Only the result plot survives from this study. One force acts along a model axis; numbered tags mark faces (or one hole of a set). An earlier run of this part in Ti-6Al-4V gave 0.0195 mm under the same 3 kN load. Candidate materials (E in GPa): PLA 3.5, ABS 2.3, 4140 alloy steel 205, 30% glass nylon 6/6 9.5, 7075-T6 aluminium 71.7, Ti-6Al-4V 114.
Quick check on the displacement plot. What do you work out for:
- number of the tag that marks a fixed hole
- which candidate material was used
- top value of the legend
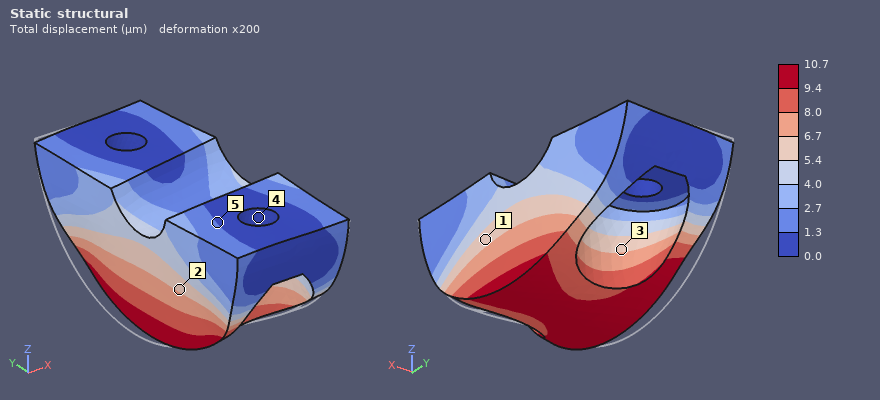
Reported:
4
4140 alloy steel
10.7 µm
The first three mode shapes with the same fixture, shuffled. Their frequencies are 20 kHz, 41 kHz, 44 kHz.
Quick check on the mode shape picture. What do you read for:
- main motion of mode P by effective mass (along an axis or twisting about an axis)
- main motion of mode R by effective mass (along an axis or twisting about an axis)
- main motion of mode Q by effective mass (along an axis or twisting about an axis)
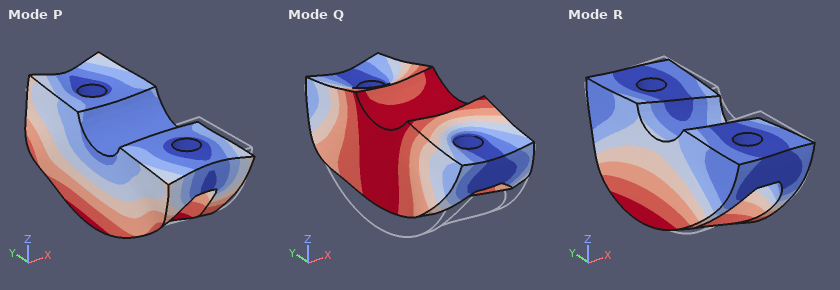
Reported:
along Y
along X
along Z
